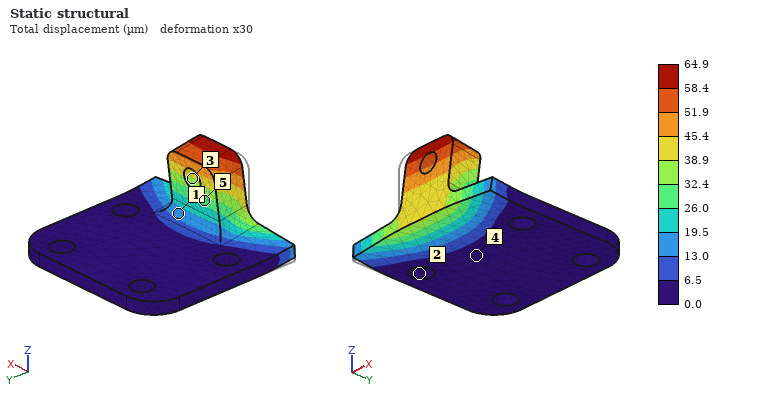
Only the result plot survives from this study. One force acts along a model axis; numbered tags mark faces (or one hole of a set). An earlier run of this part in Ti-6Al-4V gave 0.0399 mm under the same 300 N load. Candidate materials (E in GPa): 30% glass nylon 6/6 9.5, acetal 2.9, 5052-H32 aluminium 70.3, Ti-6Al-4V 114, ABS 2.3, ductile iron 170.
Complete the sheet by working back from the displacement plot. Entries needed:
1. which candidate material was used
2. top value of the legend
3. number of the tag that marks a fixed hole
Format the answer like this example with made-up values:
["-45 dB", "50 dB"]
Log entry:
["5052-H32 aluminium", "64.9 µm", "2"]
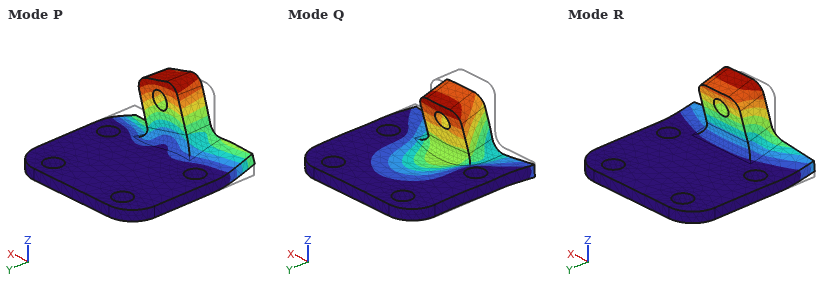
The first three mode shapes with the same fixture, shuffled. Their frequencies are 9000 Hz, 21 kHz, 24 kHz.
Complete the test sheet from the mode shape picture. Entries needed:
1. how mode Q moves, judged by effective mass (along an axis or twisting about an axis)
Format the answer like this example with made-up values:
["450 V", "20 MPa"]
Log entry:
["along Z"]
